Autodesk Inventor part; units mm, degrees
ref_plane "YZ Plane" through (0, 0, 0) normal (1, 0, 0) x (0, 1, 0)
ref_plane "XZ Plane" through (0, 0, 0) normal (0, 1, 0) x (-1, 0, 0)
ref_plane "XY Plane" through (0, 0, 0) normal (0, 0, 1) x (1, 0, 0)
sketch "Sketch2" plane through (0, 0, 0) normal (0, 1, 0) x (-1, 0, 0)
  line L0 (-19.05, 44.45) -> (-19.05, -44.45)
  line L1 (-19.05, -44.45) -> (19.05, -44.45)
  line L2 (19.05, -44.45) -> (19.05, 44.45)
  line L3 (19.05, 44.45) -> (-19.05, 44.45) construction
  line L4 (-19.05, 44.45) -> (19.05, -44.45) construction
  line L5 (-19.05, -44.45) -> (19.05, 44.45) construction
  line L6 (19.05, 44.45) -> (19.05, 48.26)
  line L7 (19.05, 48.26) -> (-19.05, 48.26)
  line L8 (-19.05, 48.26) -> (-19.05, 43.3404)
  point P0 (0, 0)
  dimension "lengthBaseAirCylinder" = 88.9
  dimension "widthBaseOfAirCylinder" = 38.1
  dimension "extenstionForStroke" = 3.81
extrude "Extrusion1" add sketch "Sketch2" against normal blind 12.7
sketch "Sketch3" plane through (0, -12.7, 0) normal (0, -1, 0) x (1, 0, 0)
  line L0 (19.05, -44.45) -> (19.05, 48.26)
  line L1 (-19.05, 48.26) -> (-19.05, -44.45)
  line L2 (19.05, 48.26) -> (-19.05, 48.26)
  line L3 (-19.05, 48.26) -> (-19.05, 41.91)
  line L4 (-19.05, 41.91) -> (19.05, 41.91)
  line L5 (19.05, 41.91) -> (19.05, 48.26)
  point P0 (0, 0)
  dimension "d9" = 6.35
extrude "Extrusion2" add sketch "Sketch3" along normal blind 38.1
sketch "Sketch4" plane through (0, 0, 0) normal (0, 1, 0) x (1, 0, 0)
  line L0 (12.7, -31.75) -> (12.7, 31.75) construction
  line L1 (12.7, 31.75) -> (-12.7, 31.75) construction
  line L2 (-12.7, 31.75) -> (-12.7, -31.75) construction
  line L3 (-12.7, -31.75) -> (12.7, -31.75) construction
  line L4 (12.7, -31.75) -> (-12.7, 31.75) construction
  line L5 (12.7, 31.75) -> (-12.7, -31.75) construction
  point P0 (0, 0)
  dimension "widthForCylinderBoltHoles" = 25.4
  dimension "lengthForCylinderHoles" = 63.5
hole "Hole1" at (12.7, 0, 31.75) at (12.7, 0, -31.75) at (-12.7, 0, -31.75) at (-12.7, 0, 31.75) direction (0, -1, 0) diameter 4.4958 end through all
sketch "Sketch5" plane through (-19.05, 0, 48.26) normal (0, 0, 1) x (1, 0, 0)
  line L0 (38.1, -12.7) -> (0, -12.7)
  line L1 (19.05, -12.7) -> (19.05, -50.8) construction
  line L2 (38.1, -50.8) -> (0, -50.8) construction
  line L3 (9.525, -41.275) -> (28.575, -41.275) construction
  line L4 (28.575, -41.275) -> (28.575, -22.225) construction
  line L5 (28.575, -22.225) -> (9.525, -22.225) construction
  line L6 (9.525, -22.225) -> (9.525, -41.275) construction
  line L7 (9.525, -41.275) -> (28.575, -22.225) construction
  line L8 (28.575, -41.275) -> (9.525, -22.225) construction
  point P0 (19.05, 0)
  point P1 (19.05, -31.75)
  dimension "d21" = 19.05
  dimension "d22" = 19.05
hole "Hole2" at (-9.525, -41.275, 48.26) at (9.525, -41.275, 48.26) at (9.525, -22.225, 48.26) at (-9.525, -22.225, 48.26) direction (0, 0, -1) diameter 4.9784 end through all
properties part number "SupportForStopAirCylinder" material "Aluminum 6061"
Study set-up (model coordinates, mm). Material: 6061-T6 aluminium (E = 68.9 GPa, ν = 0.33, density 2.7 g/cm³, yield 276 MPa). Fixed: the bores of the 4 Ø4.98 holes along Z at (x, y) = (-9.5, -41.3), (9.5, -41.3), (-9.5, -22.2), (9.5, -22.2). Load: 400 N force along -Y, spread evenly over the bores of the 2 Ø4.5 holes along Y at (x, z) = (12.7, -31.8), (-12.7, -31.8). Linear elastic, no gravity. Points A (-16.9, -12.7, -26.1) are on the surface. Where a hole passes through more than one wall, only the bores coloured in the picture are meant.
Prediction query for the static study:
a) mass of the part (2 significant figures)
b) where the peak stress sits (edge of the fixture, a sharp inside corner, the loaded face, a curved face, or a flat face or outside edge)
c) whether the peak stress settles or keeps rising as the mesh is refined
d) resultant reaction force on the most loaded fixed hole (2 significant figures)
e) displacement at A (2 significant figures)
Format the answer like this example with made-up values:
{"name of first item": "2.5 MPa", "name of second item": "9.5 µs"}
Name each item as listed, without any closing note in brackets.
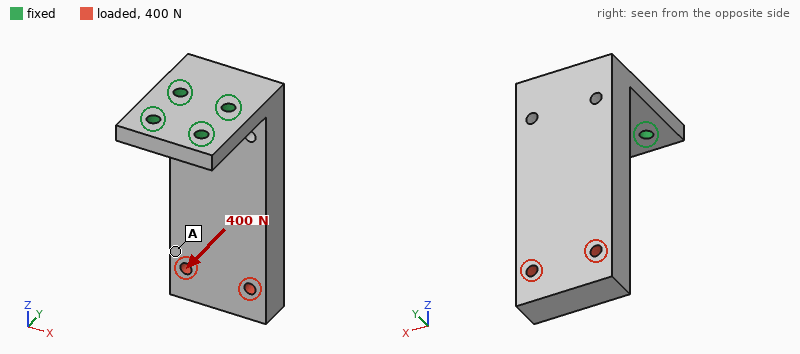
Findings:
{"mass of the part": "140 g", "where the peak stress sits": "edge of the fixture", "whether the peak stress settles or keeps rising as the mesh is refined": "keeps rising", "resultant reaction force on the most loaded fixed hole": "280 N", "displacement at A": "0.57 mm"}
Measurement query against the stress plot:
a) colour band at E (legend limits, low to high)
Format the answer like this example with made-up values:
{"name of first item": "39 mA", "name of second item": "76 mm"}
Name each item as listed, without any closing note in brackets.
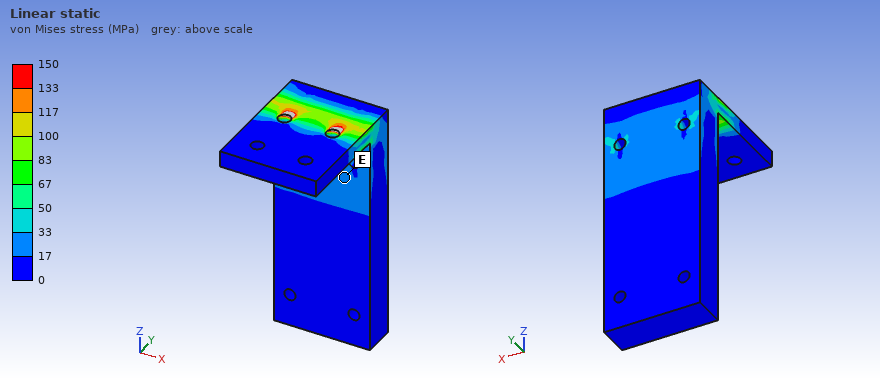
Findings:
{"colour band at E": "17 to 33 MPa"}
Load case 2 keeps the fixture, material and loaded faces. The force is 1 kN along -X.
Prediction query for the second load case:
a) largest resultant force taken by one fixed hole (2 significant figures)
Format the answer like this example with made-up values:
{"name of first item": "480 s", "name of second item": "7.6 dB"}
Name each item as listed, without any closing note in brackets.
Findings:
{"largest resultant force taken by one fixed hole": "3.3 kN"}
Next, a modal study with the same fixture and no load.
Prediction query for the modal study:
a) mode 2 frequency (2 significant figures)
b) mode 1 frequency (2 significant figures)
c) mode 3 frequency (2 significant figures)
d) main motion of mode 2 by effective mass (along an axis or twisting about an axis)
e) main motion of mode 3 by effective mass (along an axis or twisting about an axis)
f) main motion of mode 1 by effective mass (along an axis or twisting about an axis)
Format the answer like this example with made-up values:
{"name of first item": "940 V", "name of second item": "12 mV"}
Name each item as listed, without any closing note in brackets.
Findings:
{"mode 2 frequency": "1300 Hz", "mode 1 frequency": "560 Hz", "mode 3 frequency": "4400 Hz", "main motion of mode 2 by effective mass": "along X", "main motion of mode 3 by effective mass": "along Z", "main motion of mode 1 by effective mass": "along Y"}
